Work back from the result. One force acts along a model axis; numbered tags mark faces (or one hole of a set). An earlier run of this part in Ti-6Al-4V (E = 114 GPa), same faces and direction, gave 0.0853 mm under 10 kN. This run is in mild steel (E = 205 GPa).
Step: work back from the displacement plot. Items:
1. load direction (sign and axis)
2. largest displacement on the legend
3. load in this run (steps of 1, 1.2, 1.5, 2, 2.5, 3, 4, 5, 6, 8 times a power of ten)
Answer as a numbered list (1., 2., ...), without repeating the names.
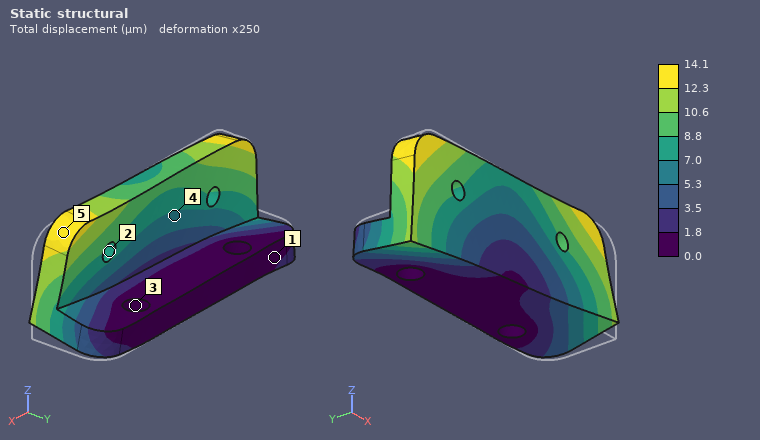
1. -X
2. 14.1 µm
3. 3 kN
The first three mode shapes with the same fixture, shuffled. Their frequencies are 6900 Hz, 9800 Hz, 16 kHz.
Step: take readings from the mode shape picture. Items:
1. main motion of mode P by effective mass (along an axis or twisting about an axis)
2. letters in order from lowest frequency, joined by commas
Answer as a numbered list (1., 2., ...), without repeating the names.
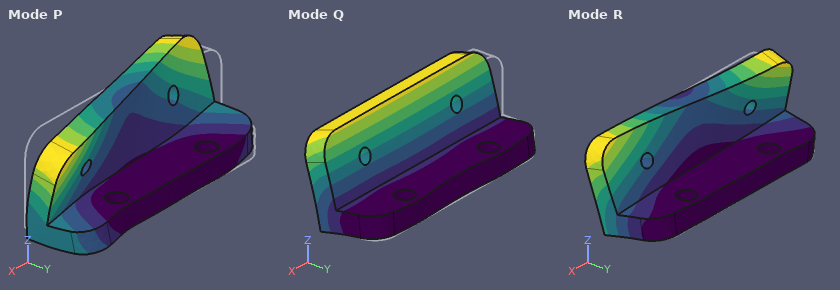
1. along X
2. Q, R, P
